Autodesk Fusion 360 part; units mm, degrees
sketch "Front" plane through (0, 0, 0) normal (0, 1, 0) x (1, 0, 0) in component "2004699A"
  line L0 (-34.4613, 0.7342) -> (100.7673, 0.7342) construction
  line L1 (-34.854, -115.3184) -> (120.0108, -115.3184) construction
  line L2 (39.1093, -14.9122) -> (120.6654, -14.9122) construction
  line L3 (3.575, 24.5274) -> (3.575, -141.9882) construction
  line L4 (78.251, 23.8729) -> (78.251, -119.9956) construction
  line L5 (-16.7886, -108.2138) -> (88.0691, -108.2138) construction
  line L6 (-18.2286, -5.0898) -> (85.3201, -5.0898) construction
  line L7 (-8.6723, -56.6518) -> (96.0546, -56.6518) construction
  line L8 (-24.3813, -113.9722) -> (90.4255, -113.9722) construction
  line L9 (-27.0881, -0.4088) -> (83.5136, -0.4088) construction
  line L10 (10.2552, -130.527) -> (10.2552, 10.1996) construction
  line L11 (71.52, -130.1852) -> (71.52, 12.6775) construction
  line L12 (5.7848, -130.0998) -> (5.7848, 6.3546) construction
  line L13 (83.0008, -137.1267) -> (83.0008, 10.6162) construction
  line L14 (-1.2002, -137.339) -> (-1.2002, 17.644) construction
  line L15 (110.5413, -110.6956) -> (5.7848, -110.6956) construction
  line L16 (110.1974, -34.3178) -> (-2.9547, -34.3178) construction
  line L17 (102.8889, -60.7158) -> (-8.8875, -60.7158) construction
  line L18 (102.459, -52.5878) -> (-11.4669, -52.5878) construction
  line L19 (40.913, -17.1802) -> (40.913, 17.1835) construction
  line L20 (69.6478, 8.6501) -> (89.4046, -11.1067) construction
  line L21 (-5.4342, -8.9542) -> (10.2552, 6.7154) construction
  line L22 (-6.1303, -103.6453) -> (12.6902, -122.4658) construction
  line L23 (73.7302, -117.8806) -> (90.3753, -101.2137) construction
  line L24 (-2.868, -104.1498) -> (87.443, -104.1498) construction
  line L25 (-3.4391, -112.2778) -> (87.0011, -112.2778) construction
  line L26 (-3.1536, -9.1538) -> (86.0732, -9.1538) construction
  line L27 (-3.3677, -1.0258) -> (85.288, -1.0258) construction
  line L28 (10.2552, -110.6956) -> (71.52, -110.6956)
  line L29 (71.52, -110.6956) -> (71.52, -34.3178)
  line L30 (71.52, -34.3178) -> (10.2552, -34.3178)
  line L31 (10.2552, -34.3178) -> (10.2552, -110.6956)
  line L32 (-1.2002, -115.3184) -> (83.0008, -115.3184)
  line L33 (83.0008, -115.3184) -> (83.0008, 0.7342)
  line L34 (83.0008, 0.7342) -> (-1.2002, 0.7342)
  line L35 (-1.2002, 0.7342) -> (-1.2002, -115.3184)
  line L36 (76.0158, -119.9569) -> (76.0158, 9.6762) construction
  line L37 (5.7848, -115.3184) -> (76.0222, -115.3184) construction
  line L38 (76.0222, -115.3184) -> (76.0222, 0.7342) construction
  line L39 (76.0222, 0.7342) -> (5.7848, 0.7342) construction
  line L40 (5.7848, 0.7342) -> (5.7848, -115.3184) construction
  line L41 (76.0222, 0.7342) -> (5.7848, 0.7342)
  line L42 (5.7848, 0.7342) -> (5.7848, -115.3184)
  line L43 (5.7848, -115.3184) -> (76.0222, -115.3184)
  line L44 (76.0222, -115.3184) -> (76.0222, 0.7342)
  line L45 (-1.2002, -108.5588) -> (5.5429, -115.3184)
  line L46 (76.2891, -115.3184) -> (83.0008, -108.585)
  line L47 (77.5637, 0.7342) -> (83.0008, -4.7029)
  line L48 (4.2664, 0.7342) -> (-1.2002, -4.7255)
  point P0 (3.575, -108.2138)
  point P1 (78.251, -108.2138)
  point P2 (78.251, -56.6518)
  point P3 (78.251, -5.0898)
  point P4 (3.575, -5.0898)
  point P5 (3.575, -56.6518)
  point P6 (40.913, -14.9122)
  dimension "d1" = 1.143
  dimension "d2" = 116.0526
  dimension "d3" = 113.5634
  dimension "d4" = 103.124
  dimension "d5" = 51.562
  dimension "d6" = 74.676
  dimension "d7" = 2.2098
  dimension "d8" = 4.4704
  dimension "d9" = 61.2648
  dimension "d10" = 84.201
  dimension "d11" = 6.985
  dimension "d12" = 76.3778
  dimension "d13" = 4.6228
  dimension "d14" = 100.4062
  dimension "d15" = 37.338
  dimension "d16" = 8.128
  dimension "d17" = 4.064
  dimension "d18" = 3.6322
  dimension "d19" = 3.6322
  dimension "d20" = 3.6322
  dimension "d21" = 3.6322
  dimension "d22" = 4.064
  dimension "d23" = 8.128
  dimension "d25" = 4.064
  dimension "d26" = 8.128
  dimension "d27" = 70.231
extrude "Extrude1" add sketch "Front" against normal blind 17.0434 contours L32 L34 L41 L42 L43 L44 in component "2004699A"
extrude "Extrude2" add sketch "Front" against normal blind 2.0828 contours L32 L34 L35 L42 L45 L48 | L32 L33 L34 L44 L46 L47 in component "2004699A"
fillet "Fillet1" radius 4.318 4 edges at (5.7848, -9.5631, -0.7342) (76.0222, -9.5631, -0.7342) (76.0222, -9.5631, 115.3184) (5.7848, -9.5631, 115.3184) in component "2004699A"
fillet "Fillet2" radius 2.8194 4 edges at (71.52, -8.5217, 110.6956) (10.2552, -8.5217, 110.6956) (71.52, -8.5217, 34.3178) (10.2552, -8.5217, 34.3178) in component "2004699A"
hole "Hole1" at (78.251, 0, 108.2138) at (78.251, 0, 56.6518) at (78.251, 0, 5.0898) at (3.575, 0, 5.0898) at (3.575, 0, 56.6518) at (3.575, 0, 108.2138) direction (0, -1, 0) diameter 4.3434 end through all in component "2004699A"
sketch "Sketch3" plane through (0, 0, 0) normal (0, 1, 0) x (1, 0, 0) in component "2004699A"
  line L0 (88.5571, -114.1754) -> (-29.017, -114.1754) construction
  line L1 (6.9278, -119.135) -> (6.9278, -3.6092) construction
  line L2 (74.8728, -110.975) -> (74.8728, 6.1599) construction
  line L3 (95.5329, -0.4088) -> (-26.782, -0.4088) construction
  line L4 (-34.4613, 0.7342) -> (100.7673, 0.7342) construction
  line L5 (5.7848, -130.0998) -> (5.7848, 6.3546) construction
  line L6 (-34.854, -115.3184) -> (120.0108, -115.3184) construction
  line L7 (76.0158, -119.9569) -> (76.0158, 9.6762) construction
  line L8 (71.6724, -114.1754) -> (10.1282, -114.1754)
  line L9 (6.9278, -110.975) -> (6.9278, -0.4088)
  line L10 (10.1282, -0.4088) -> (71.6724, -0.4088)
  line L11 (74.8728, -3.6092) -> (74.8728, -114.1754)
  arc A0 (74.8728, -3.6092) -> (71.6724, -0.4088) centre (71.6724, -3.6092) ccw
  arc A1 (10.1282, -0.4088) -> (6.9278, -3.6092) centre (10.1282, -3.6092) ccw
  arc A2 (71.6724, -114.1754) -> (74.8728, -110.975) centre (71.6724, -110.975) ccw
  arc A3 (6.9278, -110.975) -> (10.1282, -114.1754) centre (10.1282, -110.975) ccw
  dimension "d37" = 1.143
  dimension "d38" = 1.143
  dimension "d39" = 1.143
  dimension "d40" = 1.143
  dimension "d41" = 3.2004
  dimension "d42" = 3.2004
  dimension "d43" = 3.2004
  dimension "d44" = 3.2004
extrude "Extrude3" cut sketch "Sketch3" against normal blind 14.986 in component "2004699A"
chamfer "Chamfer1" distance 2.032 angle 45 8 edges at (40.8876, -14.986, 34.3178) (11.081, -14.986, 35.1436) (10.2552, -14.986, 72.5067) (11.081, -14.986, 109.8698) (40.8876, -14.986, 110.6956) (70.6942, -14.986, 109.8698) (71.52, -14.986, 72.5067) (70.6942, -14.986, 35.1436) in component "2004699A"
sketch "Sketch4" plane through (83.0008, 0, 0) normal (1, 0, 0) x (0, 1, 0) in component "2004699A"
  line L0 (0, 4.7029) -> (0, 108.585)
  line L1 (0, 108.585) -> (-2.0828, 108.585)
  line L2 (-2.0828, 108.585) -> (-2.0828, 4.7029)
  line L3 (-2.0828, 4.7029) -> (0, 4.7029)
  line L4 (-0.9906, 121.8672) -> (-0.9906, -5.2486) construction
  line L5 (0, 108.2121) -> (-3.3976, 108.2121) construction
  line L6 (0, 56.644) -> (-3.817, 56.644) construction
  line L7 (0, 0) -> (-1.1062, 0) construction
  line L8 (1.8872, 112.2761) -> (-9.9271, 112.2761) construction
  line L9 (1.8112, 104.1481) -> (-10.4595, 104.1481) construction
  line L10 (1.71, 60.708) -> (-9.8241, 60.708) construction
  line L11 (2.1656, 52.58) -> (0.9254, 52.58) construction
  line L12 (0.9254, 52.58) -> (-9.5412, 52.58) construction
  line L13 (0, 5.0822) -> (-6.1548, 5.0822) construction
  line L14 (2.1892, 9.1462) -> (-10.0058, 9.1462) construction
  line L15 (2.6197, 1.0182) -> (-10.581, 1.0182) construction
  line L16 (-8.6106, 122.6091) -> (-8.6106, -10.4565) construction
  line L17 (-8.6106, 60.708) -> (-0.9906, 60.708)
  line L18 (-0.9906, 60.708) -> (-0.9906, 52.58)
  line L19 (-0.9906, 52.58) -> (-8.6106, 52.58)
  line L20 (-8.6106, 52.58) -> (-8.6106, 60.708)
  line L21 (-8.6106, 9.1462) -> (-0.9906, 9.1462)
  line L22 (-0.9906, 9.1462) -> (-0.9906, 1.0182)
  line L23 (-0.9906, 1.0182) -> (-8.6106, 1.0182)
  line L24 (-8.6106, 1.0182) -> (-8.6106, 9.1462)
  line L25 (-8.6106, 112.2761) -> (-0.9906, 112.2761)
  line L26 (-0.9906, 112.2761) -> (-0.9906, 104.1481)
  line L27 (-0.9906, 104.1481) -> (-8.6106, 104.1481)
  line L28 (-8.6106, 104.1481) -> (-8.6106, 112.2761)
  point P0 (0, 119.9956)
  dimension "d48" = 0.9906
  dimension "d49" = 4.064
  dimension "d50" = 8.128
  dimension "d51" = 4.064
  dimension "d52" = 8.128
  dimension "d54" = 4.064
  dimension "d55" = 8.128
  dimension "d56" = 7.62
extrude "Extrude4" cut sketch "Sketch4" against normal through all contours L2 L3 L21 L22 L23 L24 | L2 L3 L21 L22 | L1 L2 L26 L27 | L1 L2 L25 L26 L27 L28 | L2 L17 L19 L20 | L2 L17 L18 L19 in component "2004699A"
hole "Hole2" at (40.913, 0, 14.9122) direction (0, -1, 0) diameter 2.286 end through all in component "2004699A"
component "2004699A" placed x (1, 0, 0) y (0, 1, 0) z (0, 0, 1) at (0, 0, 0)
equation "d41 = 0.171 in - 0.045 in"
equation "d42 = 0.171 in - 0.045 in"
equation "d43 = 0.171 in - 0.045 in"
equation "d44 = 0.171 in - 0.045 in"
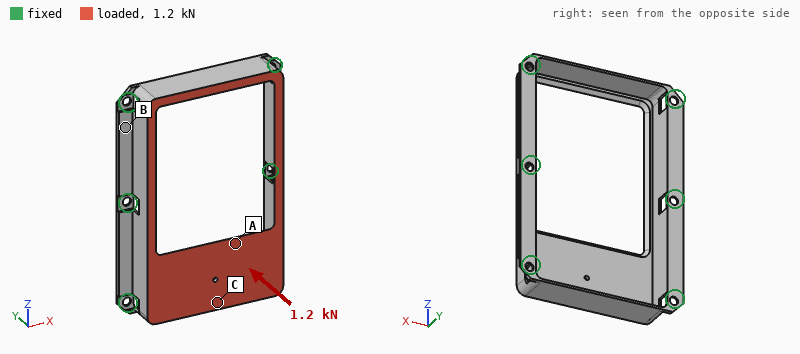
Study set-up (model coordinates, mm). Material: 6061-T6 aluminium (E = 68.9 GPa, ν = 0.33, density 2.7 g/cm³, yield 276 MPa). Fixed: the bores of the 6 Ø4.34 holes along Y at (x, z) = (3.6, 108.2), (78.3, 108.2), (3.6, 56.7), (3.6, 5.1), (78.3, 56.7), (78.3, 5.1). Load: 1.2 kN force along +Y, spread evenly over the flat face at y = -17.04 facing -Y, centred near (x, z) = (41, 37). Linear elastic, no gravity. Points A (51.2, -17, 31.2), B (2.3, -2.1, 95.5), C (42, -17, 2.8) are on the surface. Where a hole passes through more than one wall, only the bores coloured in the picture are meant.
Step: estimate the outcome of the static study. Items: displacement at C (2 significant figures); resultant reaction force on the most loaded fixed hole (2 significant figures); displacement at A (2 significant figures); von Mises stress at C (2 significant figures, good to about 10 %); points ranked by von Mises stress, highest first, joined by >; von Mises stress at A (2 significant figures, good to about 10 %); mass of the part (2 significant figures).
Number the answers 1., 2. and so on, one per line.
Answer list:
1. 0.12 mm
2. 410 N
3. 0.56 mm
4. 29 MPa
5. A > C > B
6. 97 MPa
7. 41 g
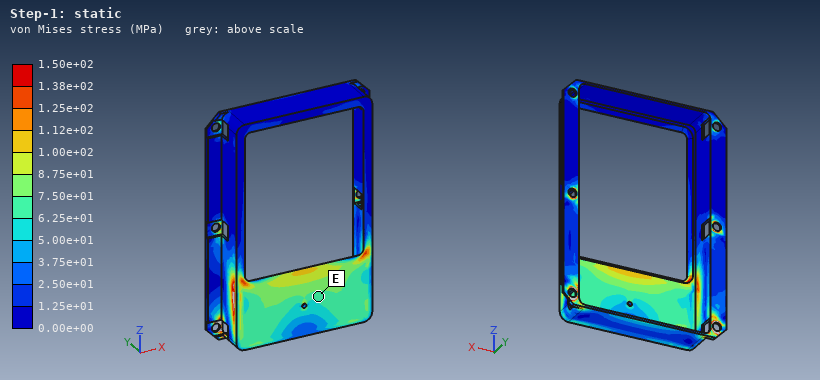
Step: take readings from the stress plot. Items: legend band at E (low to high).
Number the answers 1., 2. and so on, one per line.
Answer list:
1. 6.25e+01 to 7.50e+01 MPa
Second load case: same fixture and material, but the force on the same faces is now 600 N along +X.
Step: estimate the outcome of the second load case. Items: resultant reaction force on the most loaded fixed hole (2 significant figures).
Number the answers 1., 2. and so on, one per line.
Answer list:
1. 270 N
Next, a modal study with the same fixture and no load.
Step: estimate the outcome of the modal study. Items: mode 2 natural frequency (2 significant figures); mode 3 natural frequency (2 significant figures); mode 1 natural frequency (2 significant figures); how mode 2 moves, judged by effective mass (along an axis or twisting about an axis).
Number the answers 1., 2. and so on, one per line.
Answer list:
1. 2100 Hz
2. 3200 Hz
3. 1900 Hz
4. along Y
